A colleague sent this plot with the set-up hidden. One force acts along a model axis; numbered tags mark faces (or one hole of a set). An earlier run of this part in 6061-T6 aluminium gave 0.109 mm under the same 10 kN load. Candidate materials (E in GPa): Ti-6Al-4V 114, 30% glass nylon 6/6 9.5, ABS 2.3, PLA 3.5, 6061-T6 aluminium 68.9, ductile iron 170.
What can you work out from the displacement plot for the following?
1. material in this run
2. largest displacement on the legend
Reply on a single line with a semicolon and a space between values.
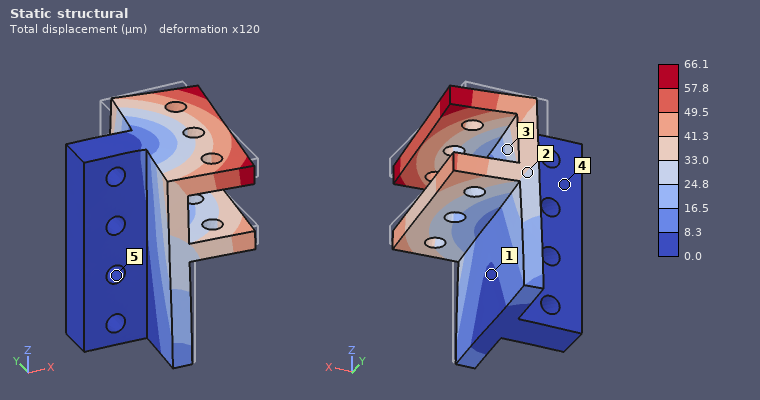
Ti-6Al-4V; 66.1 µm
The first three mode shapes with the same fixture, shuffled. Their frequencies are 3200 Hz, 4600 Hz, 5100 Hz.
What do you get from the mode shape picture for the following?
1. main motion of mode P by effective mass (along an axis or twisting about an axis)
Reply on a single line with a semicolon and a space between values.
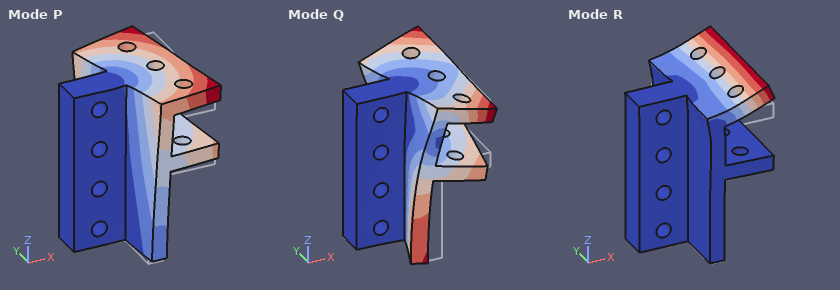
along Y
